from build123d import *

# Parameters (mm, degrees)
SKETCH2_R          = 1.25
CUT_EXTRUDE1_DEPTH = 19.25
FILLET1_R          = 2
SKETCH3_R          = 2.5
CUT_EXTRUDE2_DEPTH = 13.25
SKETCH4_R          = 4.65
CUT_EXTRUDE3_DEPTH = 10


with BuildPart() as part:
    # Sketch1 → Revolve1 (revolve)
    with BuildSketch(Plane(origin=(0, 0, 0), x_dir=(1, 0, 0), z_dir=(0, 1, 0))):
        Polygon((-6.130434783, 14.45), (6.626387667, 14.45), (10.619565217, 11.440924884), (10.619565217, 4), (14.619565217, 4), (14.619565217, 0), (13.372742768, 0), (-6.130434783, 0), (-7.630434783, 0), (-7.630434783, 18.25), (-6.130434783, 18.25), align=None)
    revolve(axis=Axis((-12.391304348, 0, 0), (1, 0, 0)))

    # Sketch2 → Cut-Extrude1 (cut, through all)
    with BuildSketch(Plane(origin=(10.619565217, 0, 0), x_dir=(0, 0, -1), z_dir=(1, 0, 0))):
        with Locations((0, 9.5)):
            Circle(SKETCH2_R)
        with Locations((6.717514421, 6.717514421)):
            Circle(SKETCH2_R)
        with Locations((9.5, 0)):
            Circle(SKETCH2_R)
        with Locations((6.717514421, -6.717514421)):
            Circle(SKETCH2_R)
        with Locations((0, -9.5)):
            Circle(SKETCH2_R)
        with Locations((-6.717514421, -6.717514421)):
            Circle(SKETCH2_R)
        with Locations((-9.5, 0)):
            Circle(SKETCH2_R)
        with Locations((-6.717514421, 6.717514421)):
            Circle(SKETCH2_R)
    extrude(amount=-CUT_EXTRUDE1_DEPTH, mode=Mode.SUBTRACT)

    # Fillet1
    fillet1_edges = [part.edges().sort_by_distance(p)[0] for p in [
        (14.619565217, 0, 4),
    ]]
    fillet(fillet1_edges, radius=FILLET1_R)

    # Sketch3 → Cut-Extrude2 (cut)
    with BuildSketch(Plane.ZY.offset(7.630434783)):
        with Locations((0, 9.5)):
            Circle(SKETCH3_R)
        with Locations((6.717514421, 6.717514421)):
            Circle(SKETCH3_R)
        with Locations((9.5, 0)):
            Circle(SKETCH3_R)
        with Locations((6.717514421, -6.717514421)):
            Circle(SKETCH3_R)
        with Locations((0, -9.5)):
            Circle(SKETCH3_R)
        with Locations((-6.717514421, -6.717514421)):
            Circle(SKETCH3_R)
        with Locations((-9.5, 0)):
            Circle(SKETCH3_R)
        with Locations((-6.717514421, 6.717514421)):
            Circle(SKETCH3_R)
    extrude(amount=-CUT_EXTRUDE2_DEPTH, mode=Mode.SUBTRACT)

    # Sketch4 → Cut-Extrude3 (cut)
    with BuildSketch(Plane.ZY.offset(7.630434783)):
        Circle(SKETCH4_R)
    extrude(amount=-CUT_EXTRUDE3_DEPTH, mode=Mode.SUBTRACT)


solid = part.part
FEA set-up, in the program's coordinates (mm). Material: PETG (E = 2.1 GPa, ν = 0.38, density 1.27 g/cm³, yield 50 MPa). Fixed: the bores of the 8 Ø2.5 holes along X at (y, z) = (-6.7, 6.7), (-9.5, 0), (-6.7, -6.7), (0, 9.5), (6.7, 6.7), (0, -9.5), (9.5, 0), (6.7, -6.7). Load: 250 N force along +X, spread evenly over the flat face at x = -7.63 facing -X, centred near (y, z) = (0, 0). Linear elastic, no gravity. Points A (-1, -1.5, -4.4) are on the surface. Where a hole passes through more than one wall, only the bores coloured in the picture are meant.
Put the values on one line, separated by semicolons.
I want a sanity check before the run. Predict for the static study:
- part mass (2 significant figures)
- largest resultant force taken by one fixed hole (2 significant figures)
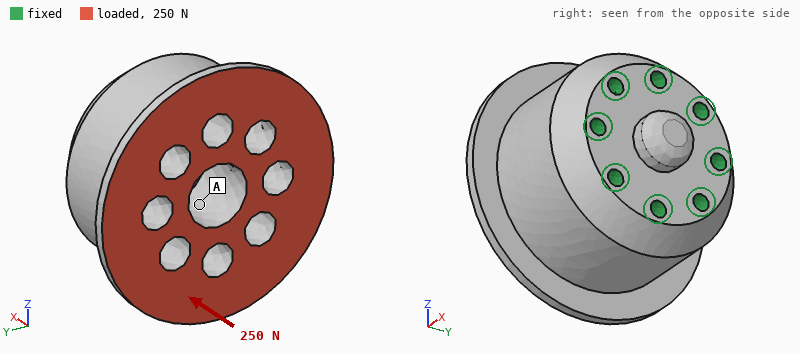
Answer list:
12 g; 31 N
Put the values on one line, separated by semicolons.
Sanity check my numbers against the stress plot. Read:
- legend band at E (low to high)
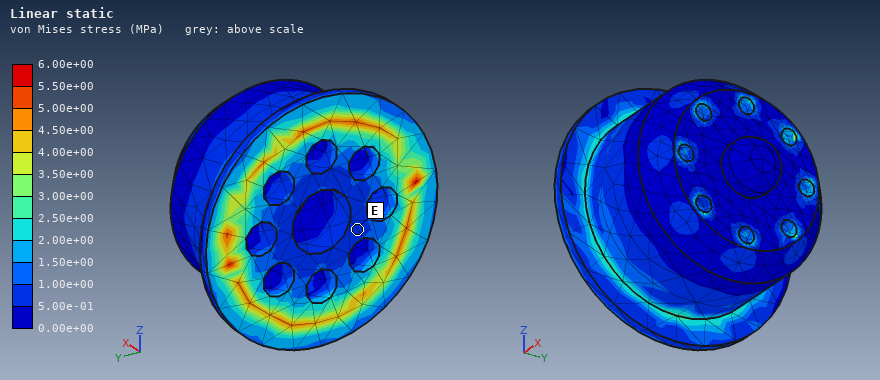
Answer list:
5.00e-01 to 1.00e+00 MPa
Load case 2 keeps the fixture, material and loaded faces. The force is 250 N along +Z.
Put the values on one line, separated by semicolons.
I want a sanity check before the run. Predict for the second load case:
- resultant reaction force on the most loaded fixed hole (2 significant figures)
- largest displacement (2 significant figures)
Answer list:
88 N; 59 µm
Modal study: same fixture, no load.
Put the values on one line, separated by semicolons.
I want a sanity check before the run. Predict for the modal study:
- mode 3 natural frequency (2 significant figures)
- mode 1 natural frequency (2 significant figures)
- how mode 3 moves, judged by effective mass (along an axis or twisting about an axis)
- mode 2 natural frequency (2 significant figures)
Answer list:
9300 Hz; 6800 Hz; twisting about X; 6800 Hz
